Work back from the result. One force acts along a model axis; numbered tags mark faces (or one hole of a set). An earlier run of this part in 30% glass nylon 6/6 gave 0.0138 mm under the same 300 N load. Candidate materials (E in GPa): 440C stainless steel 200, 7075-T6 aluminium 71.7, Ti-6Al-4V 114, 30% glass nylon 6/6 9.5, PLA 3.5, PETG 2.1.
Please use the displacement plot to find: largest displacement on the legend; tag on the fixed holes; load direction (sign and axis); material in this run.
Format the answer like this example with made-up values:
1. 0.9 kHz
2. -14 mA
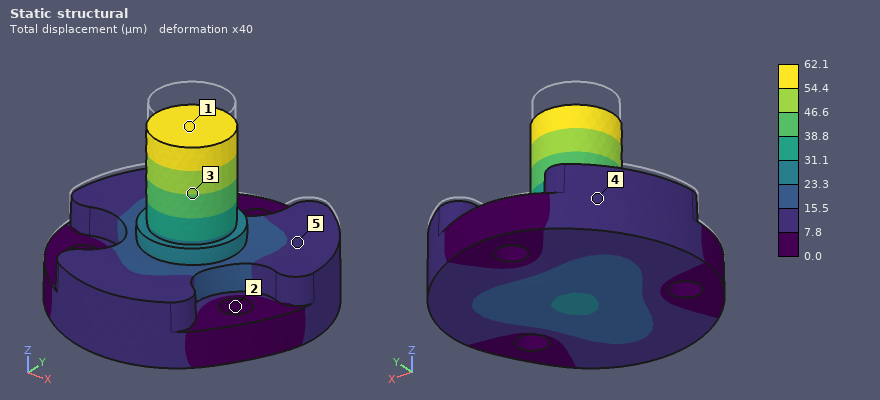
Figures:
1. 62.1 µm
2. 2
3. -Z
4. PETG
